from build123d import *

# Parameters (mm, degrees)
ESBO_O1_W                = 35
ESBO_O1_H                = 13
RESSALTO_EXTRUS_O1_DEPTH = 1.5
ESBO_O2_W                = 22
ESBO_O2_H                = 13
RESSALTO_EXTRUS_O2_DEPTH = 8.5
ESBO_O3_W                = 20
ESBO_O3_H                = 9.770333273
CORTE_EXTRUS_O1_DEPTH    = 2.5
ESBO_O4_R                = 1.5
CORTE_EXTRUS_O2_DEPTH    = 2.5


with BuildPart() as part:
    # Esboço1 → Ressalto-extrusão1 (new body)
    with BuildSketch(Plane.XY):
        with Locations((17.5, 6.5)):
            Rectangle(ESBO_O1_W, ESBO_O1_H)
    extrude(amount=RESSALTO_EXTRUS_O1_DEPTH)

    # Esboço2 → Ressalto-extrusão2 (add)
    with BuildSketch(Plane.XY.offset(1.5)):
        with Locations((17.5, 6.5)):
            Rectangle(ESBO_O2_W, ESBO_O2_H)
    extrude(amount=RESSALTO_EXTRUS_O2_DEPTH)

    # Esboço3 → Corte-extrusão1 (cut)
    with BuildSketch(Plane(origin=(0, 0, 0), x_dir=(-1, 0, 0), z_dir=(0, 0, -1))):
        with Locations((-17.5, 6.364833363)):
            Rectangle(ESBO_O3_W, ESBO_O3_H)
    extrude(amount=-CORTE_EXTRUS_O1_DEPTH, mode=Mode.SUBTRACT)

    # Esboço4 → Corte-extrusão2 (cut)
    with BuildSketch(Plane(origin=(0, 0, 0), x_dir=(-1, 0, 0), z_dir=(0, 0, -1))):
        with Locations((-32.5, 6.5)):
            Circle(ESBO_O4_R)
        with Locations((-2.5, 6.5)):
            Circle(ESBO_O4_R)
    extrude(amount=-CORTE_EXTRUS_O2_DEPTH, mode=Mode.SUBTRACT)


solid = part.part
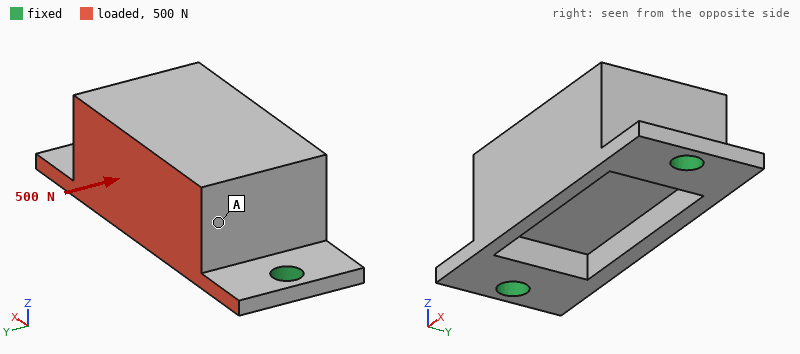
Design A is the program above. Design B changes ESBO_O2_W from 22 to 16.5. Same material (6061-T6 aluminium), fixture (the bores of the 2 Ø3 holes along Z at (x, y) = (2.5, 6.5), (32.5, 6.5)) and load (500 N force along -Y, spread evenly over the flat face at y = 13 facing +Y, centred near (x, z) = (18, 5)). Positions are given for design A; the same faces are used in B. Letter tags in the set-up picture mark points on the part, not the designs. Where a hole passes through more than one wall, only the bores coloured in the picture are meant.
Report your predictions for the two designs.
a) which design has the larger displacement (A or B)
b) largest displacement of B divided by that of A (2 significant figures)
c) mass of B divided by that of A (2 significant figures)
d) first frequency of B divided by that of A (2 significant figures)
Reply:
B
2.3
0.78
0.74
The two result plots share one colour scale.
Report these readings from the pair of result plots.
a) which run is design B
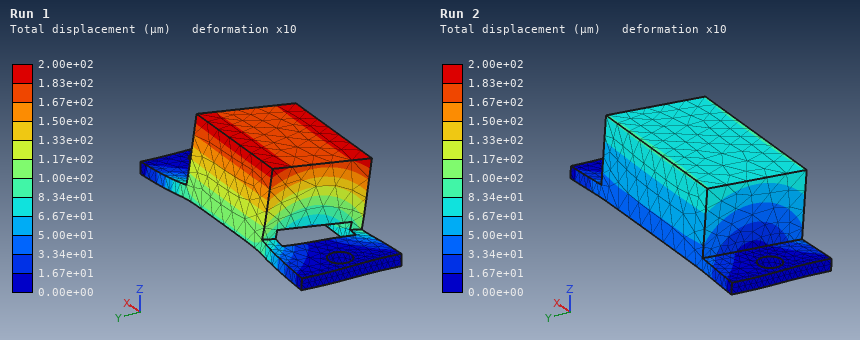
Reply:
Run 1
